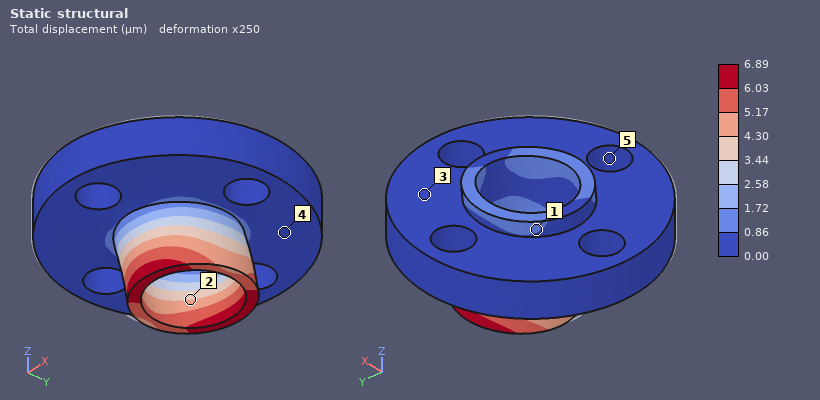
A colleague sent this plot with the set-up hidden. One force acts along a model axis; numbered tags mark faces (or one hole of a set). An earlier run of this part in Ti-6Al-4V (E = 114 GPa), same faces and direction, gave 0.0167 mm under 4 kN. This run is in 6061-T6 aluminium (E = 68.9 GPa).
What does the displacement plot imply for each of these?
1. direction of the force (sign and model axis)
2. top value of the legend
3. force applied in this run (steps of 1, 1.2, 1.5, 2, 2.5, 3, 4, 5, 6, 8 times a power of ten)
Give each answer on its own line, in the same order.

+Y
6.89 µm
1 kN
